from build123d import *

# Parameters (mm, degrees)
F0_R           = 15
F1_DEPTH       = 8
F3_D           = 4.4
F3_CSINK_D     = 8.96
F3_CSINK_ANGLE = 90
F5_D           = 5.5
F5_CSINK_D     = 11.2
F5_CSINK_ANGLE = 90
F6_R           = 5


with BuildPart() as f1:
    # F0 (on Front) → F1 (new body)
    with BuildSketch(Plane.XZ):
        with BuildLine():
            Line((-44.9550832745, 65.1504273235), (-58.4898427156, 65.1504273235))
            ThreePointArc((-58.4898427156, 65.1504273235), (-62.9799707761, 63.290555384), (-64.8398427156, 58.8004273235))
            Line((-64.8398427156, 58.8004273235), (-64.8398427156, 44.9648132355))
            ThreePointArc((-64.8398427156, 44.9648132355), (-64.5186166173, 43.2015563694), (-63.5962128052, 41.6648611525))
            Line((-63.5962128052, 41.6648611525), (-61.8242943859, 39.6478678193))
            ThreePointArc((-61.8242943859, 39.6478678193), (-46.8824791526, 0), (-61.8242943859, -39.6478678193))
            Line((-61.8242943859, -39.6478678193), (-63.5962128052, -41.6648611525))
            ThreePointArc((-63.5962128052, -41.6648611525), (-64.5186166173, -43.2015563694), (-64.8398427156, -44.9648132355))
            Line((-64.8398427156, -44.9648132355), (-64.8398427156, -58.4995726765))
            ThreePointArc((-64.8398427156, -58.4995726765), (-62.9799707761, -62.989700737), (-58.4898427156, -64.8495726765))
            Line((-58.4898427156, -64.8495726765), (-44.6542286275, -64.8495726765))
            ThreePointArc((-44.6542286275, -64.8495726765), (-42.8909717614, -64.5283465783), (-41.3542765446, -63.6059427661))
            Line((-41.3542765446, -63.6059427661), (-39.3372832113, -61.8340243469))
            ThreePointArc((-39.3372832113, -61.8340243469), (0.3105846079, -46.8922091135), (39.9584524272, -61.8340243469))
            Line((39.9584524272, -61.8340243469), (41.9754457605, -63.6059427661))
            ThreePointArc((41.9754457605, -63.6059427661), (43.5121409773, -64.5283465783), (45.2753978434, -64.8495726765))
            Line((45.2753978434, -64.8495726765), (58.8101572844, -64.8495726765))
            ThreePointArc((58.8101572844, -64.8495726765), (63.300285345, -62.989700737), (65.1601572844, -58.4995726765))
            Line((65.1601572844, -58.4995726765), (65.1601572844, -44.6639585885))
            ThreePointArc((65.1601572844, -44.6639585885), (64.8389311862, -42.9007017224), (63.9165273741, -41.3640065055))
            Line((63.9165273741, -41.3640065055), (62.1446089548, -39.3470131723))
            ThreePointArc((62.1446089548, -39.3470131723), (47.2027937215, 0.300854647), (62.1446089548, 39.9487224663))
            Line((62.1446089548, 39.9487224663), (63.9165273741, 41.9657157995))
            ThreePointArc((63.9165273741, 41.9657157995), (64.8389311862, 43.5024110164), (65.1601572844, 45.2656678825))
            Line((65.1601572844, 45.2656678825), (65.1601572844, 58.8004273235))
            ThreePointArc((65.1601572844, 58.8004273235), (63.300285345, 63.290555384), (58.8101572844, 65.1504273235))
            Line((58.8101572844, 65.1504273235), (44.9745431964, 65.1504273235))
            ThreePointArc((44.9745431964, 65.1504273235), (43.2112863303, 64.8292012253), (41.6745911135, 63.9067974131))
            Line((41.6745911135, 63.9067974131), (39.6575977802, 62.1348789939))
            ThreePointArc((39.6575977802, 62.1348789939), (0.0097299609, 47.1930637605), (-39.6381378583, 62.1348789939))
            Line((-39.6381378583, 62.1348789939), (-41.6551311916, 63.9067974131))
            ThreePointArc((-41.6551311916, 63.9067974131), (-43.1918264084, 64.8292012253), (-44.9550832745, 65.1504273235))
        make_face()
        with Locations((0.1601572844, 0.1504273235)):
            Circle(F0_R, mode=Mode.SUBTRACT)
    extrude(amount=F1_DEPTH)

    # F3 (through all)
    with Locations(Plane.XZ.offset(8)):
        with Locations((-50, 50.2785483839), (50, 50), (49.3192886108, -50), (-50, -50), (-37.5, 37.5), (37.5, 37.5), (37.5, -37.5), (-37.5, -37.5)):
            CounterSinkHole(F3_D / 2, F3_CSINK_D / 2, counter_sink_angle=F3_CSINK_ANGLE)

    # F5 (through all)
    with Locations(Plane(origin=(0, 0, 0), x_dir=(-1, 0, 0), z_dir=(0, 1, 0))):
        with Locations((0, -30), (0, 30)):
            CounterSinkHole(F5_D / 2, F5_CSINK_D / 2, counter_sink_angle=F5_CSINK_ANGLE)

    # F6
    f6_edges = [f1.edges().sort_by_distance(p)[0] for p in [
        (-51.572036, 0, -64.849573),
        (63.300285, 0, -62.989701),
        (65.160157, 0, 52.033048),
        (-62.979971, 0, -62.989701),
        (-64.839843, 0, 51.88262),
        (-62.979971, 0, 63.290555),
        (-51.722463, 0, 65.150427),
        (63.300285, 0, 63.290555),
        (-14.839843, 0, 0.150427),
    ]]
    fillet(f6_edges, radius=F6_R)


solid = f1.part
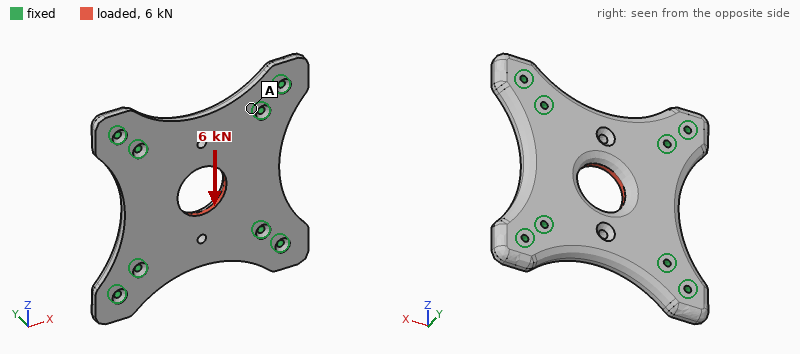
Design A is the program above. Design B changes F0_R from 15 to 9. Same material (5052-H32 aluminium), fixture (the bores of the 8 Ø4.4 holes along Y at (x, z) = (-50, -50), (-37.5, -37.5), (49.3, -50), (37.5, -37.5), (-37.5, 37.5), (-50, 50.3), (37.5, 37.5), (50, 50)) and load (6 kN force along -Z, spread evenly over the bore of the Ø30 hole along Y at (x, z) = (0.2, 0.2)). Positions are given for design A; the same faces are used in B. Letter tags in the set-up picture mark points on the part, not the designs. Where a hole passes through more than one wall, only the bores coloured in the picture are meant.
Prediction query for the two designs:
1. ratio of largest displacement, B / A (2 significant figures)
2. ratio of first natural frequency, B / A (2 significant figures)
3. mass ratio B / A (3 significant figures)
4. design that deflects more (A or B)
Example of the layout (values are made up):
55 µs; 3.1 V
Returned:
1.2; 0.96; 1.04; B
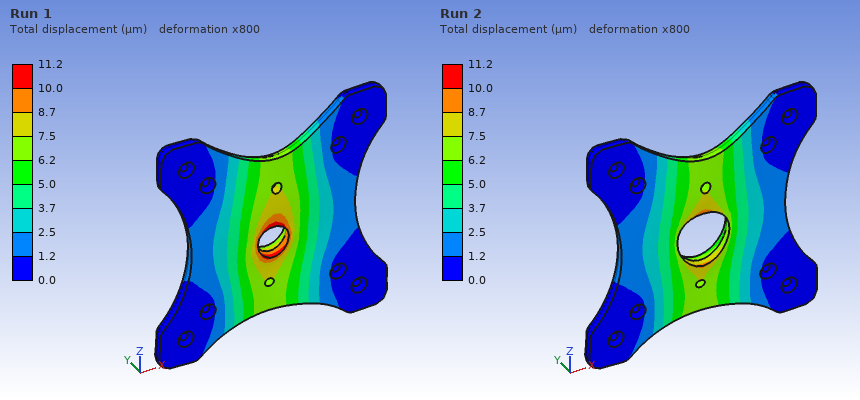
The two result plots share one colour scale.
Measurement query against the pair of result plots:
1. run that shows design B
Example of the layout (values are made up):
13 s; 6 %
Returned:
Run 1
